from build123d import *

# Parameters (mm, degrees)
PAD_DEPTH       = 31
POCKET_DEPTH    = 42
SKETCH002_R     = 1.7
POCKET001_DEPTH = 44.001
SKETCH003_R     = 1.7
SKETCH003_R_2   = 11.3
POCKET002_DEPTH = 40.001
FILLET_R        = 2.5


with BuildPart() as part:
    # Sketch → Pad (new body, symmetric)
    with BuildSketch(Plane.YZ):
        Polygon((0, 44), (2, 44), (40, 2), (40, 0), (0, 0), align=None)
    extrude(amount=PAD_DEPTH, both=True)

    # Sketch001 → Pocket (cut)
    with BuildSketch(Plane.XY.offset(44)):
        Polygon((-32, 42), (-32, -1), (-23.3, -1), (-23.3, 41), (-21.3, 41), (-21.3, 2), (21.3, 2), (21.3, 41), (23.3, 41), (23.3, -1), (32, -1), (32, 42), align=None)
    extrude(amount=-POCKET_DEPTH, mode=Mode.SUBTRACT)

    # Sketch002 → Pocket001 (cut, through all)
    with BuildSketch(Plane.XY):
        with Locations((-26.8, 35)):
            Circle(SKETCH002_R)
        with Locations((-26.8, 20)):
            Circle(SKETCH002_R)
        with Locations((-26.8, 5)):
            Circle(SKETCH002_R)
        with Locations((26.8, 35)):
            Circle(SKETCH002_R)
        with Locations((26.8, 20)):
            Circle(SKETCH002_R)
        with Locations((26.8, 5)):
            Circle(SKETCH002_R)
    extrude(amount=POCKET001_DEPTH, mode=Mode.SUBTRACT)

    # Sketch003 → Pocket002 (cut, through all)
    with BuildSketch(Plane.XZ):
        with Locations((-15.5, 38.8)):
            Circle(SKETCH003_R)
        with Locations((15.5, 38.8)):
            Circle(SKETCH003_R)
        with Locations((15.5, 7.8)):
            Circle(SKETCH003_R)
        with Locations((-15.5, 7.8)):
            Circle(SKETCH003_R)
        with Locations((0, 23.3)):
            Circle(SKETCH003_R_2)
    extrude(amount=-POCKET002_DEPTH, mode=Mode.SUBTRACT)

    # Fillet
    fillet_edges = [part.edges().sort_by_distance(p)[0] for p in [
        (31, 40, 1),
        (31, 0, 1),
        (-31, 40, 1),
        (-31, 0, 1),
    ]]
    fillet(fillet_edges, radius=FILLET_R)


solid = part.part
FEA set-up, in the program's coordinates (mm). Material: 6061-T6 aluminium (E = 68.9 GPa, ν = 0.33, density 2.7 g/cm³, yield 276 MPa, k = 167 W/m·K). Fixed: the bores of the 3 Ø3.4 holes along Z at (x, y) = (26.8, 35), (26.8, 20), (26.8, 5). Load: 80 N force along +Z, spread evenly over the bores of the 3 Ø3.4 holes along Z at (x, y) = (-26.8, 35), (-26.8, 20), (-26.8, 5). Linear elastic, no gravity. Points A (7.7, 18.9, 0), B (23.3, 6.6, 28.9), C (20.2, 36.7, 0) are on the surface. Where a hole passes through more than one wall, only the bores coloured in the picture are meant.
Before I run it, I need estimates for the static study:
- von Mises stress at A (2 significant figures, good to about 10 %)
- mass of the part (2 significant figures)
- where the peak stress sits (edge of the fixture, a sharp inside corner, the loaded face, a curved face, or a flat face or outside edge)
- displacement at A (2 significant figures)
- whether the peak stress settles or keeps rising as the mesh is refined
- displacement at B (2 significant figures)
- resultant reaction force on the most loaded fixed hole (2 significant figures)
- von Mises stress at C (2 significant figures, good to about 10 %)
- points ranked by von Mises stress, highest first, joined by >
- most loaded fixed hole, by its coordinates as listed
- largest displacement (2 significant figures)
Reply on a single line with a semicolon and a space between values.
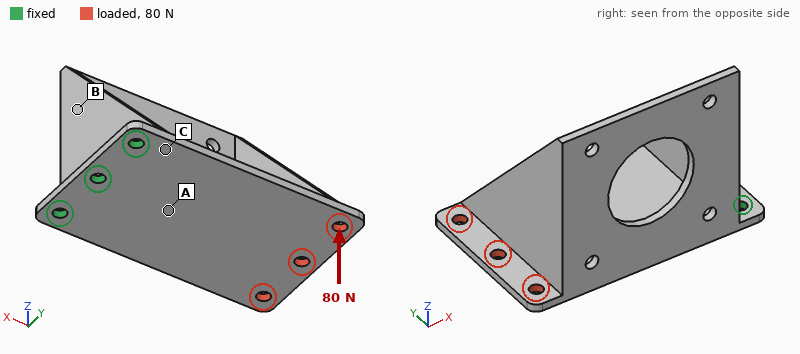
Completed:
23 MPa; 30 g; edge of the fixture; 0.20 mm; keeps rising; 0.38 mm; 66 N; 67 MPa; C > A > B; (26.8, 20); 0.98 mm
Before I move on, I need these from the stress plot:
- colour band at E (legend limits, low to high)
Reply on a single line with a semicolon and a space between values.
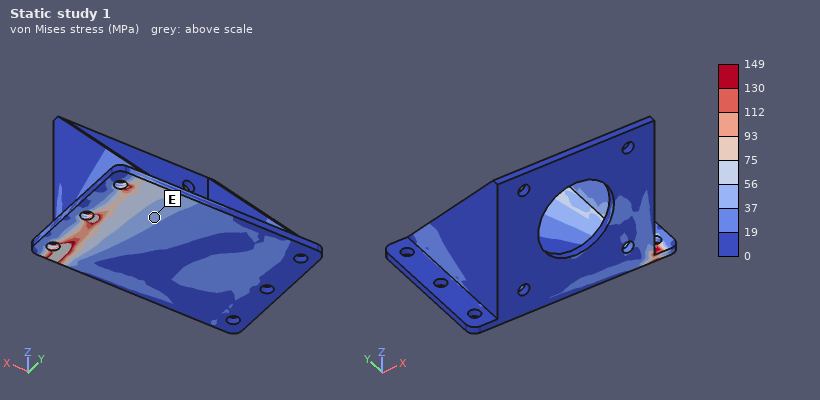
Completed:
37 to 56 MPa
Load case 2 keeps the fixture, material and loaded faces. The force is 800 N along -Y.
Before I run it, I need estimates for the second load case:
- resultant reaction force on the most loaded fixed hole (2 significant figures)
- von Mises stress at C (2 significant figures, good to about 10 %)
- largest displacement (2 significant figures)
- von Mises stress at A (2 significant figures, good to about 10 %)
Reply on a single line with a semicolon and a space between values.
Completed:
1.4 kN; 63 MPa; 0.10 mm; 26 MPa
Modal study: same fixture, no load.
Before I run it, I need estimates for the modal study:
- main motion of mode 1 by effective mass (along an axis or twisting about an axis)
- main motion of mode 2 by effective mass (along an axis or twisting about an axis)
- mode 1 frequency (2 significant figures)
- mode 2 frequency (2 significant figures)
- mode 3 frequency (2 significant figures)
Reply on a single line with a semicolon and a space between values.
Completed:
along Z; along Y; 440 Hz; 990 Hz; 3400 Hz
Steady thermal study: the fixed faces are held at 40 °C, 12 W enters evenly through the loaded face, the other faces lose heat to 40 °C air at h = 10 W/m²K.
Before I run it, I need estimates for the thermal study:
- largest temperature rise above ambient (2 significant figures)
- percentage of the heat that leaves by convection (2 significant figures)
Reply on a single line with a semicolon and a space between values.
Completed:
37 K; 16 %
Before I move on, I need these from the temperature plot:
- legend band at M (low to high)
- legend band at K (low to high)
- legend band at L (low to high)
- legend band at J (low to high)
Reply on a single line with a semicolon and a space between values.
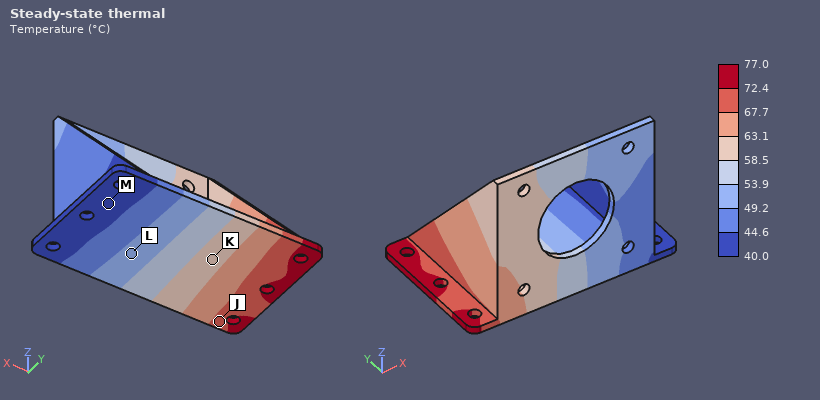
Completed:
40.0 to 44.6 °C; 58.5 to 63.1 °C; 49.2 to 53.9 °C; 67.7 to 72.4 °C
